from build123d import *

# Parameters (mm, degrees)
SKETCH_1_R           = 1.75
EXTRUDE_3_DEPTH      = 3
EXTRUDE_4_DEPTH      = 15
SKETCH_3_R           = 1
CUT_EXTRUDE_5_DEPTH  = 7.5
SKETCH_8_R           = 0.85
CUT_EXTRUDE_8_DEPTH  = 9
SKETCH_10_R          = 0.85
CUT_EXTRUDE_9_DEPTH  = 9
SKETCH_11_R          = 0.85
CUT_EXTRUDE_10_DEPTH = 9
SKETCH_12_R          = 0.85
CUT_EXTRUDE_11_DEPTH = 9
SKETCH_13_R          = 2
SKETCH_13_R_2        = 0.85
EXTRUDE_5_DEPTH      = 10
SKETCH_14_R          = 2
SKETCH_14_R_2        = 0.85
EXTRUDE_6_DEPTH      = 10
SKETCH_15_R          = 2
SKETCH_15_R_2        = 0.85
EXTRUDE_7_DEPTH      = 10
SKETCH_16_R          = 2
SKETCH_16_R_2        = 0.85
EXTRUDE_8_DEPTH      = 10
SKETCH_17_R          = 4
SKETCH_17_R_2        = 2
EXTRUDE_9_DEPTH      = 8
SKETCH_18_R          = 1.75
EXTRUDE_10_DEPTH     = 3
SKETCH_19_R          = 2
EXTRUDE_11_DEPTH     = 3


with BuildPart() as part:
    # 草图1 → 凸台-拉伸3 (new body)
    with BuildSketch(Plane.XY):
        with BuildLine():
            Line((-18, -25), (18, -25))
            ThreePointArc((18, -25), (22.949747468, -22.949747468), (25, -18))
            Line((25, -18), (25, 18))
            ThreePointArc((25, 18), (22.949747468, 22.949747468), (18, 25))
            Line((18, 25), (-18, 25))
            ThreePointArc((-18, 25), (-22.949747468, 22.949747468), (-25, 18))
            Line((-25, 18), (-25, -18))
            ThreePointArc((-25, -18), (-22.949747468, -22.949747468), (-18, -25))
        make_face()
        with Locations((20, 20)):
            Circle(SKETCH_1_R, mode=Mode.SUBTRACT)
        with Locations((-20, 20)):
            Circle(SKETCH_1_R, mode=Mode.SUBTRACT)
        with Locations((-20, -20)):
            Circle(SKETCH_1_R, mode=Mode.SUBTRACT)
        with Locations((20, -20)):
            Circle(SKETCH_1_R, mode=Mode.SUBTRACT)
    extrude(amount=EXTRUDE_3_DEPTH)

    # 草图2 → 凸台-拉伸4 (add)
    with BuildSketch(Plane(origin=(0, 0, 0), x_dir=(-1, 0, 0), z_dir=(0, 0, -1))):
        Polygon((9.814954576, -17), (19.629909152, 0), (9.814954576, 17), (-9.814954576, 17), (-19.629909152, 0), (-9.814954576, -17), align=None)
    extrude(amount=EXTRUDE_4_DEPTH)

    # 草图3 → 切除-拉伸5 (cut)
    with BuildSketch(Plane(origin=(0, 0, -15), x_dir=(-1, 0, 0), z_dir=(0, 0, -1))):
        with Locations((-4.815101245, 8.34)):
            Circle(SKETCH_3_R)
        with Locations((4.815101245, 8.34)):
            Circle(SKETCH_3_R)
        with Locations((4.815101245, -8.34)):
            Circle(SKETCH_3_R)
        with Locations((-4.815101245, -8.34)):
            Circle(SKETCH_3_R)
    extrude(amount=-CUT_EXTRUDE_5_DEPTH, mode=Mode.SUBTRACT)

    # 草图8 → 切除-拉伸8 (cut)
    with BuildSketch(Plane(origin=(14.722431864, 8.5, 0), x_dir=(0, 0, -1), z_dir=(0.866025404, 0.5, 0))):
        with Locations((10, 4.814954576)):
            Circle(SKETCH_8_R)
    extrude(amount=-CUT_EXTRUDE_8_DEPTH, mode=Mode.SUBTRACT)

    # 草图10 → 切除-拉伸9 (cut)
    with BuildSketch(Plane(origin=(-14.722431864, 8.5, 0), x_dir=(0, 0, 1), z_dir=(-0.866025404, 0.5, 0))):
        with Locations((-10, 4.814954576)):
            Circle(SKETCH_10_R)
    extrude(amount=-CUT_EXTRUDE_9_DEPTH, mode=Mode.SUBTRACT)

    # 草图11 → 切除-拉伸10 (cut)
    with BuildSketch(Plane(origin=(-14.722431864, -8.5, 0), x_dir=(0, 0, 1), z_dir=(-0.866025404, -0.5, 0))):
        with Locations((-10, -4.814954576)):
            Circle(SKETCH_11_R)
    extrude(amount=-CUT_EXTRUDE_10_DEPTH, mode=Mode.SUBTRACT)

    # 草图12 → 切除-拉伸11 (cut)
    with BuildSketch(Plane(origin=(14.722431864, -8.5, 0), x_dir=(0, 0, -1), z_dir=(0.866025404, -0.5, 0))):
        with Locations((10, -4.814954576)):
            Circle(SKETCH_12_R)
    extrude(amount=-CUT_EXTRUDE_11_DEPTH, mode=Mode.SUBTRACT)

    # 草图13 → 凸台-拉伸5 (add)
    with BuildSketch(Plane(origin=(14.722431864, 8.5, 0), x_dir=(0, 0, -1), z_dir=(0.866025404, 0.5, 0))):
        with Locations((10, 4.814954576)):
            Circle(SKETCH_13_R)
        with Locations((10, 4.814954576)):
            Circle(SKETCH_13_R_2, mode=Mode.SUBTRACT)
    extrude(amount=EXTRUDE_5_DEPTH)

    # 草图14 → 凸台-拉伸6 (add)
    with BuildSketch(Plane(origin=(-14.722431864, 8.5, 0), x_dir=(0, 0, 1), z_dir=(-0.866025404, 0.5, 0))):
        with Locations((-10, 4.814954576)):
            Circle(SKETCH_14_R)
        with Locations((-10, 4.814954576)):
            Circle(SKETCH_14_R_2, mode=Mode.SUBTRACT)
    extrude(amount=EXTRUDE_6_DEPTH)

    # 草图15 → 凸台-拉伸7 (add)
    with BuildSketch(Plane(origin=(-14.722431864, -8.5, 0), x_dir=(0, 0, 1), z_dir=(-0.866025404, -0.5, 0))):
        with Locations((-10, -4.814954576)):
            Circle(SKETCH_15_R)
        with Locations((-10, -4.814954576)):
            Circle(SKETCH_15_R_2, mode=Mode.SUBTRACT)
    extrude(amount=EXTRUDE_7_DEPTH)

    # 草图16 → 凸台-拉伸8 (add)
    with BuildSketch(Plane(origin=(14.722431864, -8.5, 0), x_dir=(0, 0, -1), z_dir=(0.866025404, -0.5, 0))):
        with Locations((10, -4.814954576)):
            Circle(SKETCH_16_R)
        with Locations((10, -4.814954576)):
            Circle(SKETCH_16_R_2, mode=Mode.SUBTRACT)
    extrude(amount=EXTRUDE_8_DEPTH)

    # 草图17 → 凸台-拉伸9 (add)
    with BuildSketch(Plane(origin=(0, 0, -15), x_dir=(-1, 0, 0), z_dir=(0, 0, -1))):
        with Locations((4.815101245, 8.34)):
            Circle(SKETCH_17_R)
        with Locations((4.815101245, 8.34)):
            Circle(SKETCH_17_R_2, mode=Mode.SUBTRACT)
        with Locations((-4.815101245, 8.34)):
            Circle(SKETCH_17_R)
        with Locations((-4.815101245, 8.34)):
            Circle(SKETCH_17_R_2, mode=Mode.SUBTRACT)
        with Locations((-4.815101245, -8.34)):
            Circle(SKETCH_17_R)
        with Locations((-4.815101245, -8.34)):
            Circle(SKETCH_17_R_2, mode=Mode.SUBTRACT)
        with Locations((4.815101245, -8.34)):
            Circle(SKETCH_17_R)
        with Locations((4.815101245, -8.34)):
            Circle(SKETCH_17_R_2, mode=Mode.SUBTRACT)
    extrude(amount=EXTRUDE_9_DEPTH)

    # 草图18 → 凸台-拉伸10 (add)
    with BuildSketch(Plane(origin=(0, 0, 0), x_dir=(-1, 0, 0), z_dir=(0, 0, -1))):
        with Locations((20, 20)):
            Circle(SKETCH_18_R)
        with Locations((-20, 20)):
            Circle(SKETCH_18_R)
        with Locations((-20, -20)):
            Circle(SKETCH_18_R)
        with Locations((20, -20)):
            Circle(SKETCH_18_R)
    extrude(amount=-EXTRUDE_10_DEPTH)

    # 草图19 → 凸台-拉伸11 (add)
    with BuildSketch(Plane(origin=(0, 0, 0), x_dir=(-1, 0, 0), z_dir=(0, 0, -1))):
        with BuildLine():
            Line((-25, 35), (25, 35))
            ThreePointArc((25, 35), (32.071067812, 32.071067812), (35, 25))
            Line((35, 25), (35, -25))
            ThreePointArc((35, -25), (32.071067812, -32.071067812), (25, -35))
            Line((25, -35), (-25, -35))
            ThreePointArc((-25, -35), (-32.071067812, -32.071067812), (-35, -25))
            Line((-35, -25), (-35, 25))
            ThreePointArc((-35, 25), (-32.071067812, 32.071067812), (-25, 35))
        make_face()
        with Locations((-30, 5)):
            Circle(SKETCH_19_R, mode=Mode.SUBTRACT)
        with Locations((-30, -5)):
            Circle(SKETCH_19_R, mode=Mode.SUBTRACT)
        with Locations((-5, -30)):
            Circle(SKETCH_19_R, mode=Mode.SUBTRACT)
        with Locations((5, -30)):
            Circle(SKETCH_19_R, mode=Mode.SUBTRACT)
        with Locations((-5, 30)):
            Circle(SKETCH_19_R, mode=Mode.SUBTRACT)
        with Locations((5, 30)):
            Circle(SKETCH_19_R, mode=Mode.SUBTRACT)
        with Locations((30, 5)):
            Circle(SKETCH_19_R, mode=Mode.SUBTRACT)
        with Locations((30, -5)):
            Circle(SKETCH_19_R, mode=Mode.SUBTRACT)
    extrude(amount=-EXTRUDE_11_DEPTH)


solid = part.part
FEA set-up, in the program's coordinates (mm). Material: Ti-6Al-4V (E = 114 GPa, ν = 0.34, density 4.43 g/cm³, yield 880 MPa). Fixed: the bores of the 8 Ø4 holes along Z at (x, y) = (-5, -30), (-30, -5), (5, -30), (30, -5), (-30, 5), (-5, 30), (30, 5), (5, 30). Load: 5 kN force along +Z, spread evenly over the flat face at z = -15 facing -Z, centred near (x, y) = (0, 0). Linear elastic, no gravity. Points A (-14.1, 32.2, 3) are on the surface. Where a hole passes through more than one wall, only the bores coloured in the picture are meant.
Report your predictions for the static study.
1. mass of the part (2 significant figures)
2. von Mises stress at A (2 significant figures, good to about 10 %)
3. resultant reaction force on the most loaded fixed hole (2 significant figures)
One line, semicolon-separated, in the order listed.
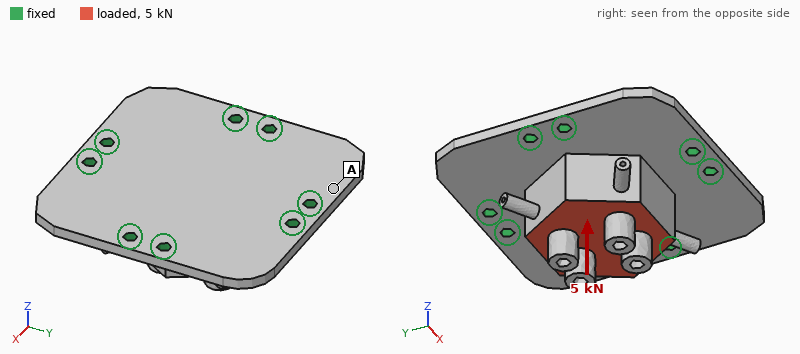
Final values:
140 g; 22 MPa; 730 N
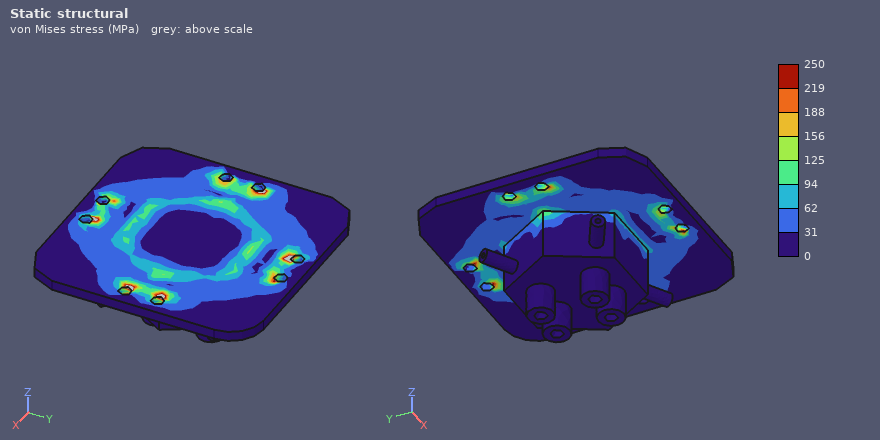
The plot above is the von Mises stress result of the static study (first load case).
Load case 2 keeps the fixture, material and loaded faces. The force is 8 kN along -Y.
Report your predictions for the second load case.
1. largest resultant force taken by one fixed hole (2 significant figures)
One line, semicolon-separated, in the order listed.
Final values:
2.0 kN
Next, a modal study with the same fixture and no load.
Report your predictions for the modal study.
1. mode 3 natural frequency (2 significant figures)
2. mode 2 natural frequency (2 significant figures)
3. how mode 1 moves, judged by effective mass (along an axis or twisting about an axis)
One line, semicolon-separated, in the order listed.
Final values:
6600 Hz; 6500 Hz; along Z
